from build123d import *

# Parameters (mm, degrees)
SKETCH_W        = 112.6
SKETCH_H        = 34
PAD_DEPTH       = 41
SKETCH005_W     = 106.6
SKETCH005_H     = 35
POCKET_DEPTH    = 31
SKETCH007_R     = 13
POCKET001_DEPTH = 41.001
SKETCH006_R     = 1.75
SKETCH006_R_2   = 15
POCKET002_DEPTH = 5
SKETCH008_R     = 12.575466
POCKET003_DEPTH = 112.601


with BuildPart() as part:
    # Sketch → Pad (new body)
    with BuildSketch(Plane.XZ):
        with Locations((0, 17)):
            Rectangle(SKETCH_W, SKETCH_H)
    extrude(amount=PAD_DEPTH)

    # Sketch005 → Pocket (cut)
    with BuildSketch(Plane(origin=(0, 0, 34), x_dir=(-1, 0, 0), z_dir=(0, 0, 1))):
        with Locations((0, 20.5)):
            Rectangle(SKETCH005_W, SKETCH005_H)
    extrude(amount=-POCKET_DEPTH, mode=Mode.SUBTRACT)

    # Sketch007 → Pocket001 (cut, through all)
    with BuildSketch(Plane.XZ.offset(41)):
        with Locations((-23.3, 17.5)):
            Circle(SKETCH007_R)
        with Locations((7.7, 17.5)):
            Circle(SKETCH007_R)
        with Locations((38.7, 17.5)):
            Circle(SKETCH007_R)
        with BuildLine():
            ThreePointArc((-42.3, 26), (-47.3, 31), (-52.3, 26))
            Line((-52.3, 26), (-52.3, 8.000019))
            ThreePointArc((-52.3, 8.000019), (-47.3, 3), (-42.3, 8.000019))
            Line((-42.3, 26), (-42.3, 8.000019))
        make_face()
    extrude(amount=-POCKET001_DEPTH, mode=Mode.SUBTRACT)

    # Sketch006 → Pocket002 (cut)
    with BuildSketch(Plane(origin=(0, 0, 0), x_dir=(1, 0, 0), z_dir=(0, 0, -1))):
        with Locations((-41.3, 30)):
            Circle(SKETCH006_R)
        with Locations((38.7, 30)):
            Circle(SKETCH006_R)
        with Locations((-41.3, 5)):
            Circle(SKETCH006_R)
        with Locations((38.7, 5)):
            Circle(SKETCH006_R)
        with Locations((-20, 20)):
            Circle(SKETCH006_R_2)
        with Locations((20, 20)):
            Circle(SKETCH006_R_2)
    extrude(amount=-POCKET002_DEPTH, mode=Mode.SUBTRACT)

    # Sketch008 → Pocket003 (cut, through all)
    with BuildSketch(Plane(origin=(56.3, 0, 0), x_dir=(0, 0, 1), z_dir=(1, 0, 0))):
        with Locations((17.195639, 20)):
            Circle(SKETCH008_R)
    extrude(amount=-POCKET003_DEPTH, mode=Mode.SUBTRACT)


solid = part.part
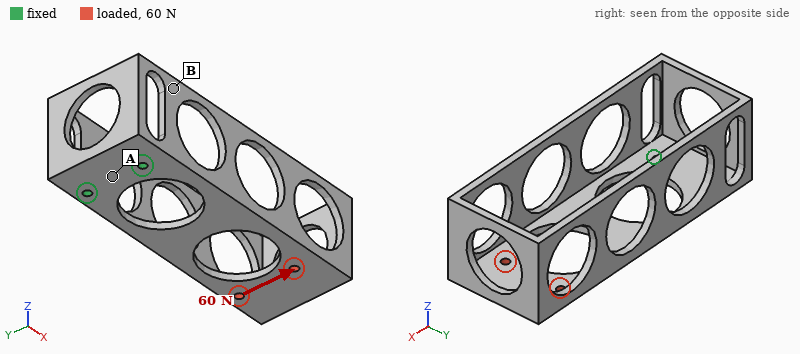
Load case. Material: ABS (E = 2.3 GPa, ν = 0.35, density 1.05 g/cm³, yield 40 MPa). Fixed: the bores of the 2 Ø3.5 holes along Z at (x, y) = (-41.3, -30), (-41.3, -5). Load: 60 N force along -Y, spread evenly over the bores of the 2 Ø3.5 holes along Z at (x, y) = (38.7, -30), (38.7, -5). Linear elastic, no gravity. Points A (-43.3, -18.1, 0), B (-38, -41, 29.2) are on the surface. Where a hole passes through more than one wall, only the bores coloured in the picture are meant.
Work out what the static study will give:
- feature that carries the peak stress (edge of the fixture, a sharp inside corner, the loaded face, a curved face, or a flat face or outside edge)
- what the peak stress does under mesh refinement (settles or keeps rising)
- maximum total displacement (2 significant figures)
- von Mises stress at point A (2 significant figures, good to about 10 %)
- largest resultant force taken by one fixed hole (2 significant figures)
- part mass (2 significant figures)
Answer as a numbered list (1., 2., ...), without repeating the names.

1. edge of the fixture
2. keeps rising
3. 1.2 mm
4. 2.8 MPa
5. 180 N
6. 24 g
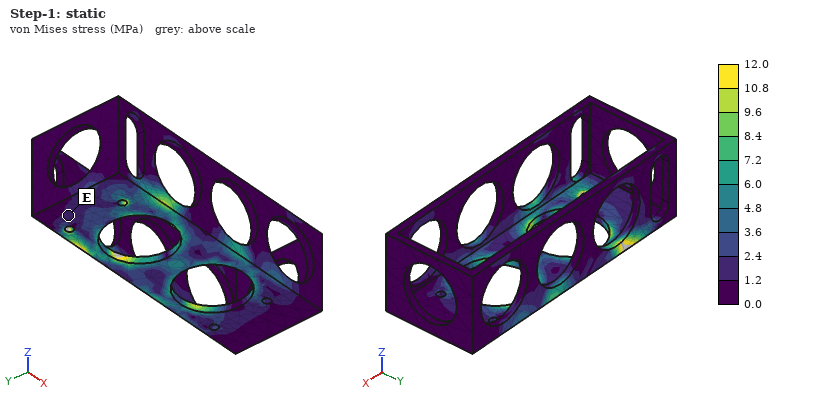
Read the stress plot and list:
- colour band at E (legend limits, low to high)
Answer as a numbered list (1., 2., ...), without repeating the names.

1. 1.2 to 2.4 MPa
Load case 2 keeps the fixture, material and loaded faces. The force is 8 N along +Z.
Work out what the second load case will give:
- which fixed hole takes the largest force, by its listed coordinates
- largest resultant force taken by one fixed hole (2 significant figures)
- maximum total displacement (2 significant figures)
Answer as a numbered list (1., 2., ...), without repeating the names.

1. (-41.3, -5)
2. 6.2 N
3. 1.3 mm
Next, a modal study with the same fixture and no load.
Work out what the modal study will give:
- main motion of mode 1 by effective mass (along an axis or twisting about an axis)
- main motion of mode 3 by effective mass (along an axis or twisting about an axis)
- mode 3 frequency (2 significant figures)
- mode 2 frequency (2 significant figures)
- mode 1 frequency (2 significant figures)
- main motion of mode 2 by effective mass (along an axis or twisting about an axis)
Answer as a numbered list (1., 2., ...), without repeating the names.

1. along Z
2. along Y
3. 460 Hz
4. 200 Hz
5. 130 Hz
6. along Y
